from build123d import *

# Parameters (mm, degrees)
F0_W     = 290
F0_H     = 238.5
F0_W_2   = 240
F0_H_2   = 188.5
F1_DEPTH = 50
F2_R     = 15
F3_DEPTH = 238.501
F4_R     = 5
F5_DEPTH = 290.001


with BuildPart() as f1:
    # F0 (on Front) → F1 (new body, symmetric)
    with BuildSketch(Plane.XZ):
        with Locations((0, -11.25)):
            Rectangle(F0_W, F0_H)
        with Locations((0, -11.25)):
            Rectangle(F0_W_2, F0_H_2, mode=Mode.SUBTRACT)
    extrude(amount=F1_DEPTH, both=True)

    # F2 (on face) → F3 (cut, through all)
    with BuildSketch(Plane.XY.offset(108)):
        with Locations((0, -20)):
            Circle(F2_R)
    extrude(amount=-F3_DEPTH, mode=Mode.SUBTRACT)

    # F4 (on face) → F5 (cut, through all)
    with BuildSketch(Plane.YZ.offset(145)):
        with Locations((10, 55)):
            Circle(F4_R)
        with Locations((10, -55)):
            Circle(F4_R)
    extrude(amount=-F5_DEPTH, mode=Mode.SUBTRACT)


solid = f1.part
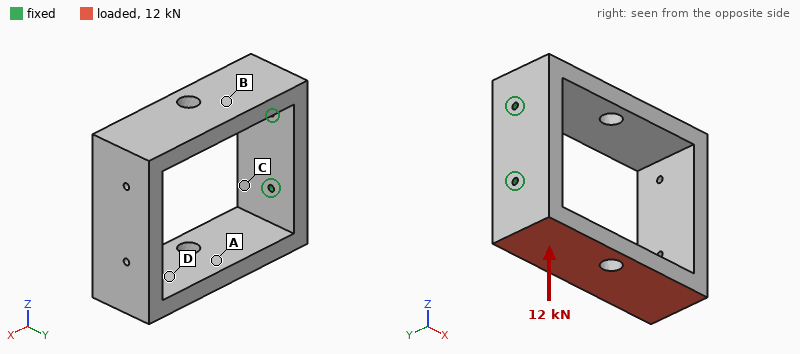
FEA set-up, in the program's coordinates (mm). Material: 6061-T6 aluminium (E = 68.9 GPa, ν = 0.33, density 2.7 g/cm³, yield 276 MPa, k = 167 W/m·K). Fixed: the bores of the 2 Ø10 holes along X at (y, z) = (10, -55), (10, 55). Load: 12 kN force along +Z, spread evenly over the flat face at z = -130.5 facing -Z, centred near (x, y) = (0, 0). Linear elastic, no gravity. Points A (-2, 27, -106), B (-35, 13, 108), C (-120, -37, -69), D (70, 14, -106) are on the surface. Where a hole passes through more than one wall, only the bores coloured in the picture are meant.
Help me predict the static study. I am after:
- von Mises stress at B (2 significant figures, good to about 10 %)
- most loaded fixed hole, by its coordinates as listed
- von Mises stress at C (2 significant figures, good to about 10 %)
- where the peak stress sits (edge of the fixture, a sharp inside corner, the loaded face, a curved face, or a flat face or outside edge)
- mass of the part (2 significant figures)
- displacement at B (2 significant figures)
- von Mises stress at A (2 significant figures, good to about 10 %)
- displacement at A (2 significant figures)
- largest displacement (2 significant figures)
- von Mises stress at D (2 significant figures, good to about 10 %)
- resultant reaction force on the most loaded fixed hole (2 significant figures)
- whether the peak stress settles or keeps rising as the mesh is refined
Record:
15 MPa
(10, -55)
51 MPa
edge of the fixture
6.3 kg
0.42 mm
25 MPa
0.79 mm
1.3 mm
30 MPa
11 kN
keeps rising
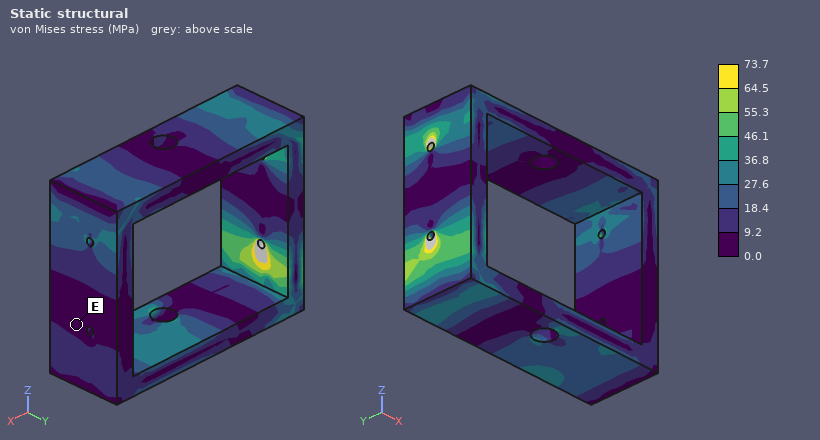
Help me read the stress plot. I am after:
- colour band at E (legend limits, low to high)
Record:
0.0 to 9.2 MPa
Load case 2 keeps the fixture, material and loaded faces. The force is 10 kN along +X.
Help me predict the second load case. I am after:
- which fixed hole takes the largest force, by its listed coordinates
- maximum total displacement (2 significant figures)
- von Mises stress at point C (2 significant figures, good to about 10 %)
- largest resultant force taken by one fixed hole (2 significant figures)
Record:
(10, -55)
0.39 mm
26 MPa
13 kN
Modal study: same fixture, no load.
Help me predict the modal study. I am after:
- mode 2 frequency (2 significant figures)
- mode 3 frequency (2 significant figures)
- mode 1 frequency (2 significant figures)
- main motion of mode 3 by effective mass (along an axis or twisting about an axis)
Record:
220 Hz
490 Hz
210 Hz
twisting about X
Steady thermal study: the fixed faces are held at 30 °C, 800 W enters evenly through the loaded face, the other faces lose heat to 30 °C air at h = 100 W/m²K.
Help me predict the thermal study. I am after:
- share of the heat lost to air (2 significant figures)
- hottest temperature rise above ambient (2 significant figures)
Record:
71 %
86 K
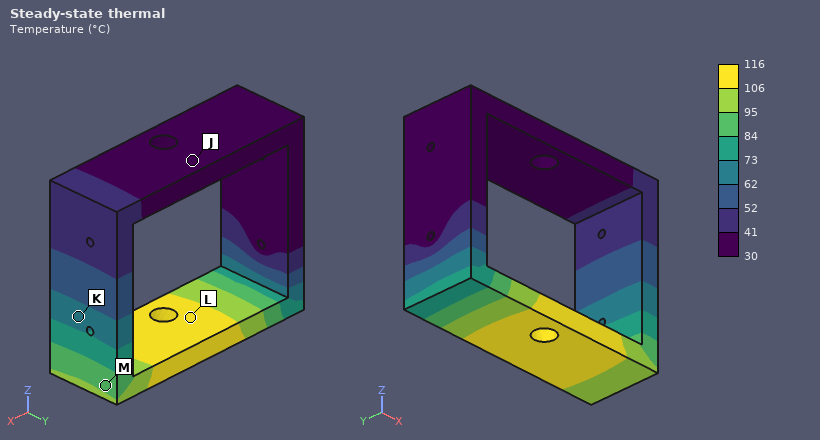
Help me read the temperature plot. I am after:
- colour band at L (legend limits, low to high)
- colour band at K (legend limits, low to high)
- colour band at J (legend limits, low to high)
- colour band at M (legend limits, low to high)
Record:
106 to 116 °C
62 to 73 °C
30 to 41 °C
84 to 95 °C
